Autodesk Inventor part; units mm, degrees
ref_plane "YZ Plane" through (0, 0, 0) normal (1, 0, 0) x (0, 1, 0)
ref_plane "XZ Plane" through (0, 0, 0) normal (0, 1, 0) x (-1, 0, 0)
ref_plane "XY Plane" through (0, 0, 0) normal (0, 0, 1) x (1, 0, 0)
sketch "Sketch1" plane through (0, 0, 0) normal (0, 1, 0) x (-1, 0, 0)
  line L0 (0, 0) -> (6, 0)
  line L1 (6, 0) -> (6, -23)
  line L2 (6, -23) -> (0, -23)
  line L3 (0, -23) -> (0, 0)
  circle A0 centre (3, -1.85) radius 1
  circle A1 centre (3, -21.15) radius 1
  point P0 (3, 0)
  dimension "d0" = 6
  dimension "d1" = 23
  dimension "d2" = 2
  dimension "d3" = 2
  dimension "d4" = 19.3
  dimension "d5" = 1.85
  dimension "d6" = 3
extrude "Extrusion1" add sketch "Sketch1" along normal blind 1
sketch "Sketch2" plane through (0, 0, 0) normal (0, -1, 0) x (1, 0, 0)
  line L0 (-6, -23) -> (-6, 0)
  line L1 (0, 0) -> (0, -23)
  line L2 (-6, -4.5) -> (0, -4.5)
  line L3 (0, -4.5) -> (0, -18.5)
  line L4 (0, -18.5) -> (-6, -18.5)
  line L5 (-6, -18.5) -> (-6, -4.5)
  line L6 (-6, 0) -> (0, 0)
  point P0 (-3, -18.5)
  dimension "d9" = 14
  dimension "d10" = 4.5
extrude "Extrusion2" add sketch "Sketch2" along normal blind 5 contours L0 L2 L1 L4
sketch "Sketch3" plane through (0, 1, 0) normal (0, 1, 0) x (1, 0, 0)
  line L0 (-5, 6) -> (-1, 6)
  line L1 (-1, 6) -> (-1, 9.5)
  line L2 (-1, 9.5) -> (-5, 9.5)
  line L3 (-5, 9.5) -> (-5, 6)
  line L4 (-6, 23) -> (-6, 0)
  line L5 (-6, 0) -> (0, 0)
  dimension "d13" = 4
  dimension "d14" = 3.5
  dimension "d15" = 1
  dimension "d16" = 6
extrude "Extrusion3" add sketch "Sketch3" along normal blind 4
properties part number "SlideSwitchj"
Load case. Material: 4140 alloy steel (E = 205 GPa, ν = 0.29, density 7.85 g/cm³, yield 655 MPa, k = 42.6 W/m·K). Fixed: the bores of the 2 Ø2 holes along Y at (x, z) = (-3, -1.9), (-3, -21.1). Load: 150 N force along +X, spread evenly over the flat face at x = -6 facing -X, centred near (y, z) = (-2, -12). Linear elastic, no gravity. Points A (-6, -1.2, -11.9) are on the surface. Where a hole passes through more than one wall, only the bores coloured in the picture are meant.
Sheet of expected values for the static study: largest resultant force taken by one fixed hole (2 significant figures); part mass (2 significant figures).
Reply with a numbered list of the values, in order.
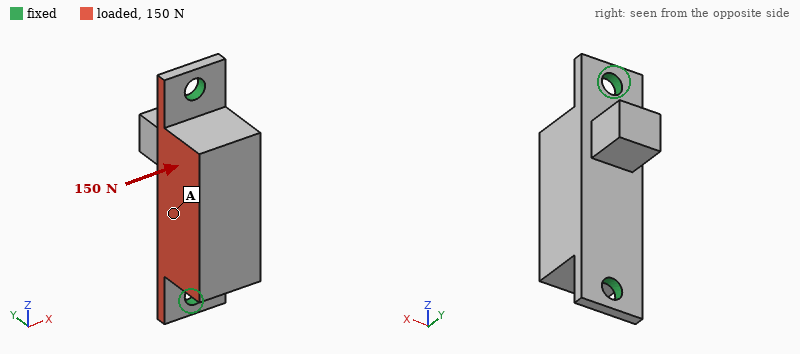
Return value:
1. 75 N
2. 4.8 g
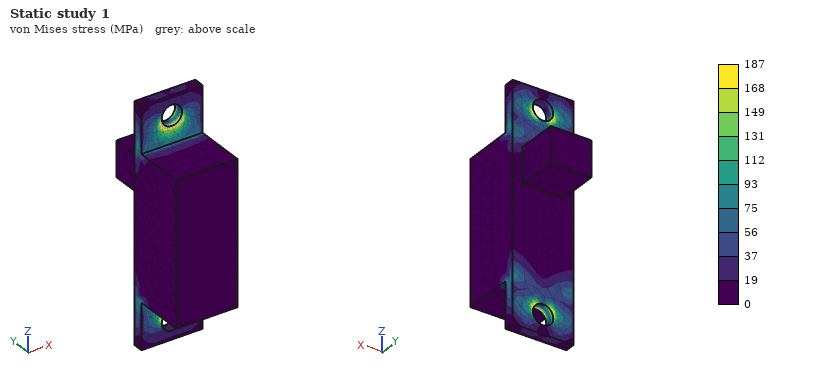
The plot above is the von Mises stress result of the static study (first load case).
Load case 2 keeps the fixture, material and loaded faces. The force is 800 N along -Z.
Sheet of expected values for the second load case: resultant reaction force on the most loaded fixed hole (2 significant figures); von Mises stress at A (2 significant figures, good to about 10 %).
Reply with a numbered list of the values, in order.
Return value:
1. 440 N
2. 27 MPa
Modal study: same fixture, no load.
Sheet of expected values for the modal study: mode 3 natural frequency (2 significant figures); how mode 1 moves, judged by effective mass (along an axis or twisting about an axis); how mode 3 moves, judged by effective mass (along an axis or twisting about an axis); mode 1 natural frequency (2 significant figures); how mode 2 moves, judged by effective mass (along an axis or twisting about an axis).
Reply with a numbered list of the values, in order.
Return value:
1. 33 kHz
2. along X
3. along X
4. 9600 Hz
5. along Y
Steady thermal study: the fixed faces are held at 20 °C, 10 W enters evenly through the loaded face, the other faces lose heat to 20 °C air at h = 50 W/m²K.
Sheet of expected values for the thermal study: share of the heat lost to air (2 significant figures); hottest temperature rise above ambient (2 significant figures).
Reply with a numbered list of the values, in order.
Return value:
1. 11 %
2. 67 K
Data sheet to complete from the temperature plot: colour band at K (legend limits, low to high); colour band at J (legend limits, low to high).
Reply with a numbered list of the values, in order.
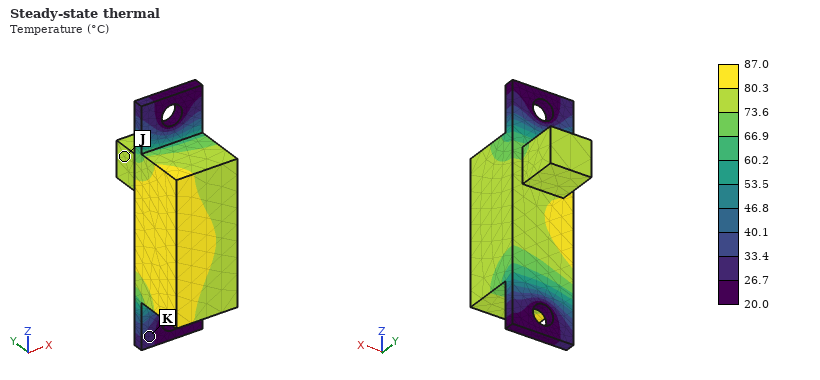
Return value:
1. 26.7 to 33.4 °C
2. 73.6 to 80.3 °C
